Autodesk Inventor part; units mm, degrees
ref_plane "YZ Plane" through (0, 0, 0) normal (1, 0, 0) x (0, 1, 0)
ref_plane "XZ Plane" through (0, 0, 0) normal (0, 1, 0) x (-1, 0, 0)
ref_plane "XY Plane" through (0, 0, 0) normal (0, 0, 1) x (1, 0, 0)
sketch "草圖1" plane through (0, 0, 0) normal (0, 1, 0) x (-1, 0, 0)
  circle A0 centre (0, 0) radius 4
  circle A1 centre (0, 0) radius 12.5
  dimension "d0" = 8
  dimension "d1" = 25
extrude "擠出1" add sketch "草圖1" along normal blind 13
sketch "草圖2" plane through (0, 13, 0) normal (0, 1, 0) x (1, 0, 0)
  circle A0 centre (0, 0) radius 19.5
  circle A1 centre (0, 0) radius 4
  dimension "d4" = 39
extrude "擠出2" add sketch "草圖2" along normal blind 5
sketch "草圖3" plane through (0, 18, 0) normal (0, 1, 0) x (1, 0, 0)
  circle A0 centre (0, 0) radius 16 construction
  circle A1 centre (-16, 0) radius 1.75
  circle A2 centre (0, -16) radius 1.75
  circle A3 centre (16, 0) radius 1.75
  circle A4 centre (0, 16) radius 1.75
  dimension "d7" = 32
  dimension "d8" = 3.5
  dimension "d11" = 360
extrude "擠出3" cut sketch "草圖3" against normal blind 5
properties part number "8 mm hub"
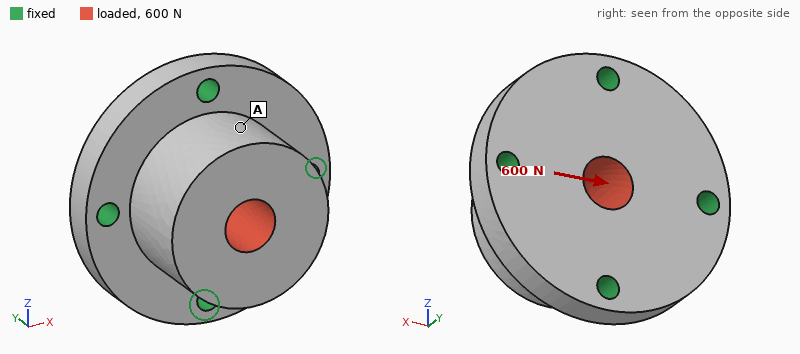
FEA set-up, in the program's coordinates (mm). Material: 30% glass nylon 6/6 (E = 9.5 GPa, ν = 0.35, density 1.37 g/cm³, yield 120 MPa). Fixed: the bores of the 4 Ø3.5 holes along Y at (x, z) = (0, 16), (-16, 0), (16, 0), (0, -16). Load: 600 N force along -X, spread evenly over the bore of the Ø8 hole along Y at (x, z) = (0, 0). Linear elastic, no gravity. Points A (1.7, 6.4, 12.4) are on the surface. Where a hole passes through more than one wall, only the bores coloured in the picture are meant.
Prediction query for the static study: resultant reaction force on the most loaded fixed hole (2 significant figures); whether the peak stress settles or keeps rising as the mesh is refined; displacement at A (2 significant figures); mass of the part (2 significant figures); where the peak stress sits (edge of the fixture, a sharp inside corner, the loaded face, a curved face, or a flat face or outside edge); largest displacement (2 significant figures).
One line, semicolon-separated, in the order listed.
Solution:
230 N; keeps rising; 6.3 µm; 15 g; edge of the fixture; 11 µm
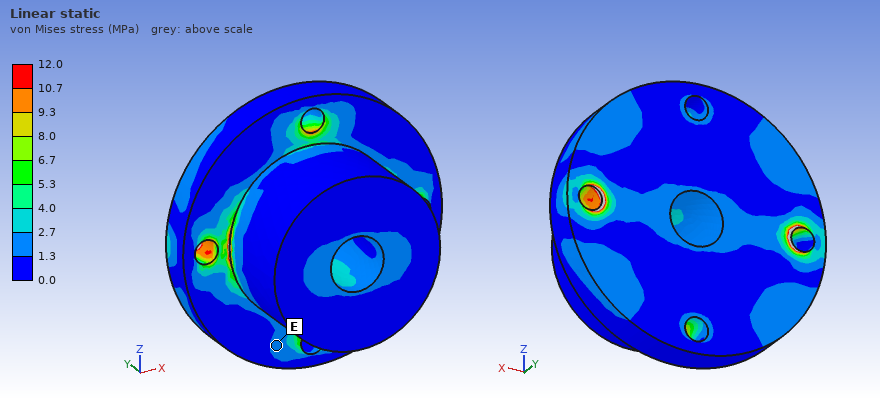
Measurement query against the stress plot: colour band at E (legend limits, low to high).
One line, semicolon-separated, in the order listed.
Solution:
1.3 to 2.7 MPa
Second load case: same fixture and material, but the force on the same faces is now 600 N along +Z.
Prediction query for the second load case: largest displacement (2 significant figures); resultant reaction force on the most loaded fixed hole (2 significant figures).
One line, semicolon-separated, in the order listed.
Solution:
11 µm; 230 N
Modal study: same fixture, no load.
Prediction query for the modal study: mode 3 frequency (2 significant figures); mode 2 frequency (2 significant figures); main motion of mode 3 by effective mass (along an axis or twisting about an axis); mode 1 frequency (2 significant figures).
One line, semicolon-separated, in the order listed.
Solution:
14 kHz; 12 kHz; along Y; 12 kHz
